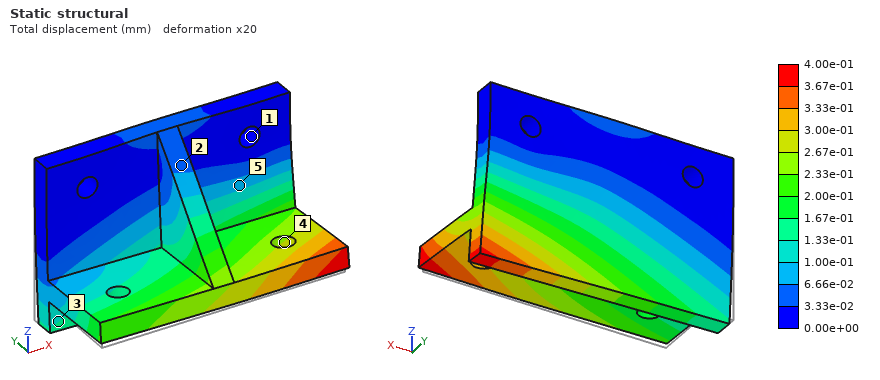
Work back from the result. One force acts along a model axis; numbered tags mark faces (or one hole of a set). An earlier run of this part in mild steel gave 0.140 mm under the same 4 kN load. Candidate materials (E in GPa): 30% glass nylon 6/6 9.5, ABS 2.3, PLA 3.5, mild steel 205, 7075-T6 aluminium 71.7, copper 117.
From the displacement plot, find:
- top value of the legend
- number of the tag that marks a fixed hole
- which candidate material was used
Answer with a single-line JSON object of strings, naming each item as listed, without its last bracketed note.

{"top value of the legend": "4.00e-01 mm", "number of the tag that marks a fixed hole": "1", "which candidate material was used": "7075-T6 aluminium"}
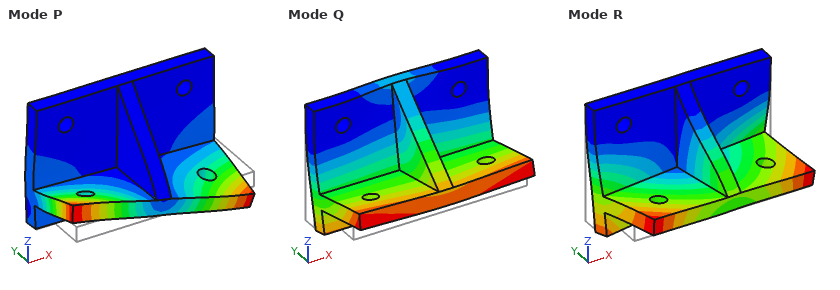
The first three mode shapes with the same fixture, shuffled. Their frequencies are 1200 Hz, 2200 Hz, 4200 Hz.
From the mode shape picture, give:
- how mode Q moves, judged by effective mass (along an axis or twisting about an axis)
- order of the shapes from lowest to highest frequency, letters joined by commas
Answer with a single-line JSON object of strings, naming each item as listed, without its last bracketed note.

{"how mode Q moves, judged by effective mass": "along Y", "order of the shapes from lowest to highest frequency, letters joined by commas": "Q, R, P"}
